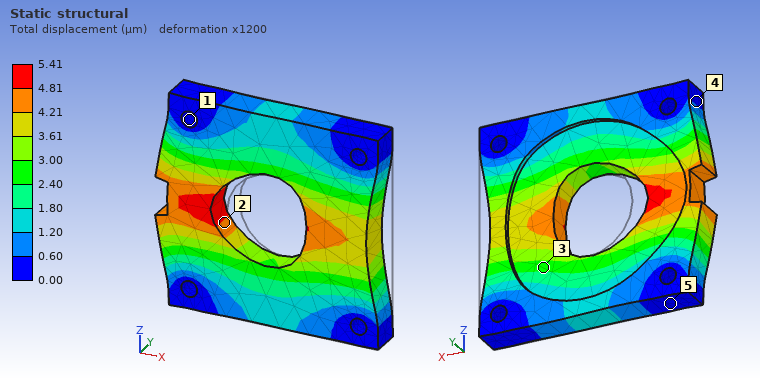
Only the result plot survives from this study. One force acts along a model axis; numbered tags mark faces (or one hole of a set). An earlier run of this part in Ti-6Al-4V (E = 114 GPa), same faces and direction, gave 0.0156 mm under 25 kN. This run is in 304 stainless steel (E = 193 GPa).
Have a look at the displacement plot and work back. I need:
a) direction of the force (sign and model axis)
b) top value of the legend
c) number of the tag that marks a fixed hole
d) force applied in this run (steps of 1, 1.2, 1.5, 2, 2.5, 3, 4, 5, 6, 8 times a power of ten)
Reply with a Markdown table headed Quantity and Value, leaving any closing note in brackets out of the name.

| Quantity | Value |
|---|---|
| direction of the force | -X |
| top value of the legend | 5.41 µm |
| number of the tag that marks a fixed hole | 1 |
| force applied in this run | 15 kN |
